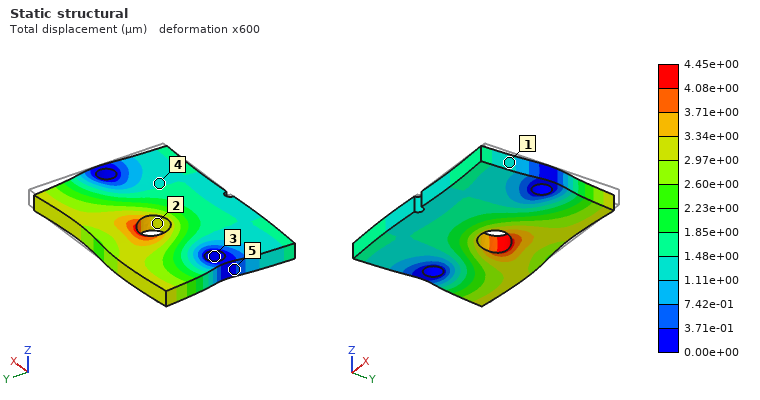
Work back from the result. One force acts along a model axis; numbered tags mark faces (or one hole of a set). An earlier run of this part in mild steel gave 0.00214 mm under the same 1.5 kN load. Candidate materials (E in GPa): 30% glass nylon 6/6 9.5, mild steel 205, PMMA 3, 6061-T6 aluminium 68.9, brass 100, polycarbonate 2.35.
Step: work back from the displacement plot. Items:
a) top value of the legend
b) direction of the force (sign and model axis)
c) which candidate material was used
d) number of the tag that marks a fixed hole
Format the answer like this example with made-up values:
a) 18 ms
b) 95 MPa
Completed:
a) 4.45e+00 µm
b) -X
c) brass
d) 3
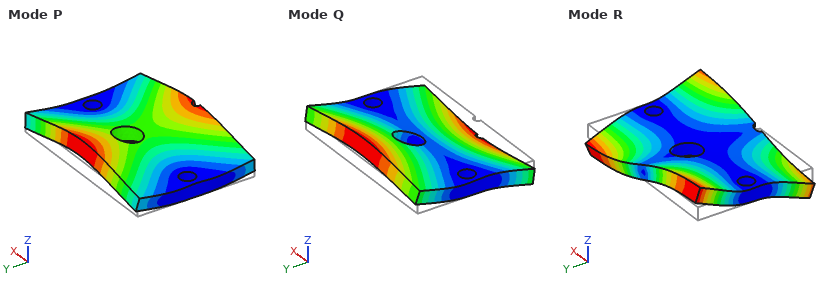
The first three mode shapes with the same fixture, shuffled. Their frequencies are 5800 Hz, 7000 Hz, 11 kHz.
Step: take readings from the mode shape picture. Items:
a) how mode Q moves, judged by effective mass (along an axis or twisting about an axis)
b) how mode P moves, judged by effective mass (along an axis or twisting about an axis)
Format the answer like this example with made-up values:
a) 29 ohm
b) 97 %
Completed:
a) twisting about X
b) along Z
